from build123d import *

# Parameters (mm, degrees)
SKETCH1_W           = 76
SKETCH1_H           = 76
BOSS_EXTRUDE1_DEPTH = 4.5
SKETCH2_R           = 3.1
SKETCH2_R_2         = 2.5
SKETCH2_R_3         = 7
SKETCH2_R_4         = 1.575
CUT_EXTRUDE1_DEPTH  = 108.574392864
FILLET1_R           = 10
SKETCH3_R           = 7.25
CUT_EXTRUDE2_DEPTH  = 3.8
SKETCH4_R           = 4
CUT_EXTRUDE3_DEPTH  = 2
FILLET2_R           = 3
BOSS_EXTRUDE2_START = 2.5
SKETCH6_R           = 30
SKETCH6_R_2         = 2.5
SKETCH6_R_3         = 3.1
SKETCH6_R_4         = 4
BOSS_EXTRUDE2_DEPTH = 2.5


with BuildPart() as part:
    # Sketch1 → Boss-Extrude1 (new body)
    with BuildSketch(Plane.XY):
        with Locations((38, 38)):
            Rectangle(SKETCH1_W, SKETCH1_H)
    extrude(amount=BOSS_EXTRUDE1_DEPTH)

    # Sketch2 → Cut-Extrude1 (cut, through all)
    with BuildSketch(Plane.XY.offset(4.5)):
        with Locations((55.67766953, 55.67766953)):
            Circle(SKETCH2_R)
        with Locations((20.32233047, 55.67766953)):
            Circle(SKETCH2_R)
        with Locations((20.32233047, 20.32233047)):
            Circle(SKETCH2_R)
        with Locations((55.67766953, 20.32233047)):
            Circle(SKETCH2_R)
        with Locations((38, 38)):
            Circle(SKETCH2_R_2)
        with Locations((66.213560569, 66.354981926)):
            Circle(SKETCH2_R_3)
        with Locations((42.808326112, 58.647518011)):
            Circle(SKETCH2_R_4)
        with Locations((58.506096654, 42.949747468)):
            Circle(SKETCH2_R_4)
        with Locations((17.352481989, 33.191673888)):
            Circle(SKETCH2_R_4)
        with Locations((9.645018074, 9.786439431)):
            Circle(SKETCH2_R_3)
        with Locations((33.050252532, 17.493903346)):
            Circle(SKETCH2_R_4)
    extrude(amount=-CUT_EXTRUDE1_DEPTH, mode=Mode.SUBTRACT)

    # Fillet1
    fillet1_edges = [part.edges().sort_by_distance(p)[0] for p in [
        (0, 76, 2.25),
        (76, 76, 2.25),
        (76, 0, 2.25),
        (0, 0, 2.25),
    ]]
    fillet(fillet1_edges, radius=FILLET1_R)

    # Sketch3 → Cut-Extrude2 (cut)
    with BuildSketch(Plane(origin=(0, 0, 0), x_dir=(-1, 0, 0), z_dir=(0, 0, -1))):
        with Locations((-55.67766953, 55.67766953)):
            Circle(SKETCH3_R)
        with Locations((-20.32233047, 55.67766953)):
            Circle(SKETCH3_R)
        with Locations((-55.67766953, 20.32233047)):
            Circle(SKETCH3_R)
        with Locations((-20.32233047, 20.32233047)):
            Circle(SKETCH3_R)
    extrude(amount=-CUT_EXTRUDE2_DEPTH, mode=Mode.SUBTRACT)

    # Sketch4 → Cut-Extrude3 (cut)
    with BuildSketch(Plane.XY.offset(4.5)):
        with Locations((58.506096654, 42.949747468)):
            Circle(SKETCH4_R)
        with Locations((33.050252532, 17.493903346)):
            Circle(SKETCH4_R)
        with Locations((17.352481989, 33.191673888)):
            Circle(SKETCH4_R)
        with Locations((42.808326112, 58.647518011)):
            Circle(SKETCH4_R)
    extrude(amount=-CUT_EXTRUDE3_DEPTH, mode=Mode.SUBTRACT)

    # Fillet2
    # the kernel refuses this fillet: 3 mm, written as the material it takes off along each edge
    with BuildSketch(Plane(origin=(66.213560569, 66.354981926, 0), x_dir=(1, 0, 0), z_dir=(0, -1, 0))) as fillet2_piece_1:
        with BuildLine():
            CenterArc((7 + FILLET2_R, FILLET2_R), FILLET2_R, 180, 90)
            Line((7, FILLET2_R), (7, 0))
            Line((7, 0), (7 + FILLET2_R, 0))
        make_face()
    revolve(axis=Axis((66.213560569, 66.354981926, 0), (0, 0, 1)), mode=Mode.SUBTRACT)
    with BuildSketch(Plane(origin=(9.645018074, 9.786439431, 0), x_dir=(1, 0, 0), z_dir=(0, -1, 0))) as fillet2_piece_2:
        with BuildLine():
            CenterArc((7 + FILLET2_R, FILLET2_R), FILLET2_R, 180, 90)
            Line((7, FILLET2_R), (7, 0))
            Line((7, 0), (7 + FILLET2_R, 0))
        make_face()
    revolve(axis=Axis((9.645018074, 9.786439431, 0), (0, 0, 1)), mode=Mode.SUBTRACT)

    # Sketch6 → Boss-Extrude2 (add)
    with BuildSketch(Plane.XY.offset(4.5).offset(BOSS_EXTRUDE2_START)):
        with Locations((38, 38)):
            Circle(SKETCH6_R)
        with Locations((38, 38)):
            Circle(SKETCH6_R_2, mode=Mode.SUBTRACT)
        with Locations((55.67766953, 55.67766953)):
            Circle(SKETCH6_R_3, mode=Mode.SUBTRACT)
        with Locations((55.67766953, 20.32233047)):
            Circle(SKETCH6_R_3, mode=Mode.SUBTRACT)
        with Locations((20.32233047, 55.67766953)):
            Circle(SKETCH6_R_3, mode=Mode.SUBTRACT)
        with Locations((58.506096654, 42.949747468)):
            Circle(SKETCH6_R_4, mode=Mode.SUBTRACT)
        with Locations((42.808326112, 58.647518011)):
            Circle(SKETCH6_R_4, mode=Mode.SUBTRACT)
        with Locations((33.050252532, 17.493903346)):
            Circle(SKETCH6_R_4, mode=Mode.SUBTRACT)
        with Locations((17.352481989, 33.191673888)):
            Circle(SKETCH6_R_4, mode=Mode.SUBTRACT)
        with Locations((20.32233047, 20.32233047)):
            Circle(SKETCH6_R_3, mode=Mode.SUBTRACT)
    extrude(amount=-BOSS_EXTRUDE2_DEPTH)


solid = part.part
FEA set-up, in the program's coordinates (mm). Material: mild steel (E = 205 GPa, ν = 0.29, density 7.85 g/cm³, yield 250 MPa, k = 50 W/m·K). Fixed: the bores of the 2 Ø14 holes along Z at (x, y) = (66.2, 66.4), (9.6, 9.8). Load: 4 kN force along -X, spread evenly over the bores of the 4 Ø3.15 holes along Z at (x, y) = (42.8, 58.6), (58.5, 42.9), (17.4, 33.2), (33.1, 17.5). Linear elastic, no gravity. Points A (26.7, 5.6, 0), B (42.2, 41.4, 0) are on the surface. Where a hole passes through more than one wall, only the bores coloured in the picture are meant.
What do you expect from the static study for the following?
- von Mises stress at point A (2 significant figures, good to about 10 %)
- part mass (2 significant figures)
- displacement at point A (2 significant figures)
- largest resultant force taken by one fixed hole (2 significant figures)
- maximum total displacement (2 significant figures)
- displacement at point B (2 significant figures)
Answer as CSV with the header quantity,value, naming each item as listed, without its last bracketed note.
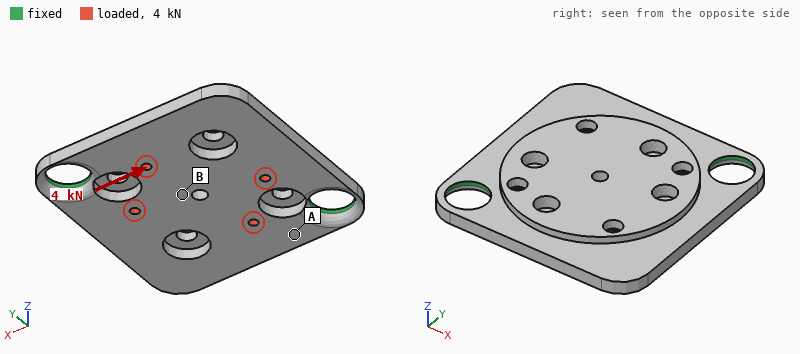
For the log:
quantity,value
von Mises stress at point A,19 MPa
part mass,210 g
displacement at point A,7.6 µm
largest resultant force taken by one fixed hole,2.0 kN
maximum total displacement,33 µm
displacement at point B,5.7 µm
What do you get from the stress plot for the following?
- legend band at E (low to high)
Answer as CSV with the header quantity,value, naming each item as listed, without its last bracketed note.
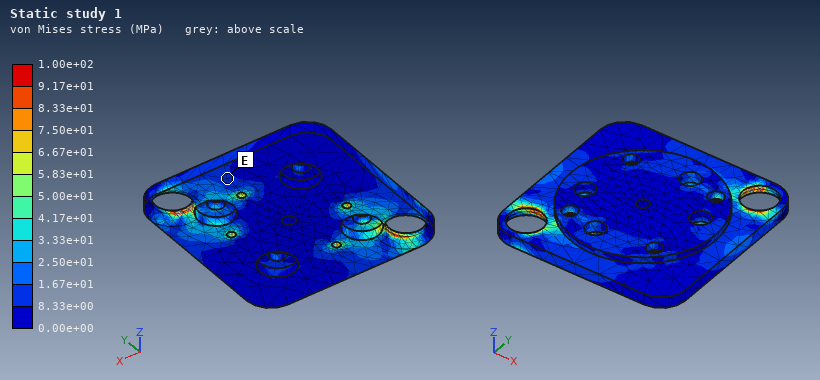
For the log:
quantity,value
legend band at E,8.33e+00 to 1.67e+01 MPa
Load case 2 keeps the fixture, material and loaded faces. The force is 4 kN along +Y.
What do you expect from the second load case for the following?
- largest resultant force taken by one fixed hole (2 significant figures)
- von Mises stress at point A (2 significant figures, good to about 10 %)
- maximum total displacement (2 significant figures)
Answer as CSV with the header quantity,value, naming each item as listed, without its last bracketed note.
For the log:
quantity,value
largest resultant force taken by one fixed hole,2.0 kN
von Mises stress at point A,19 MPa
maximum total displacement,33 µm
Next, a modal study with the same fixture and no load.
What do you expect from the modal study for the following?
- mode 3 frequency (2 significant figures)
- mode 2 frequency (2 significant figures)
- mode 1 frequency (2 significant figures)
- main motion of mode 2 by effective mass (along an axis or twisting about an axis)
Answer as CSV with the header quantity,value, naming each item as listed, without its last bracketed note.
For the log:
quantity,value
mode 3 frequency,6300 Hz
mode 2 frequency,2300 Hz
mode 1 frequency,1500 Hz
main motion of mode 2 by effective mass,along Z
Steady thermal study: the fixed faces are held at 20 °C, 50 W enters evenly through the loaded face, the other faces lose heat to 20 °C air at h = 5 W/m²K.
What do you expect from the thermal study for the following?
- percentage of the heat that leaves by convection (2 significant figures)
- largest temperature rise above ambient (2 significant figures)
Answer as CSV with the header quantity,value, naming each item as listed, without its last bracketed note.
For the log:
quantity,value
percentage of the heat that leaves by convection,7.3 %
largest temperature rise above ambient,86 K
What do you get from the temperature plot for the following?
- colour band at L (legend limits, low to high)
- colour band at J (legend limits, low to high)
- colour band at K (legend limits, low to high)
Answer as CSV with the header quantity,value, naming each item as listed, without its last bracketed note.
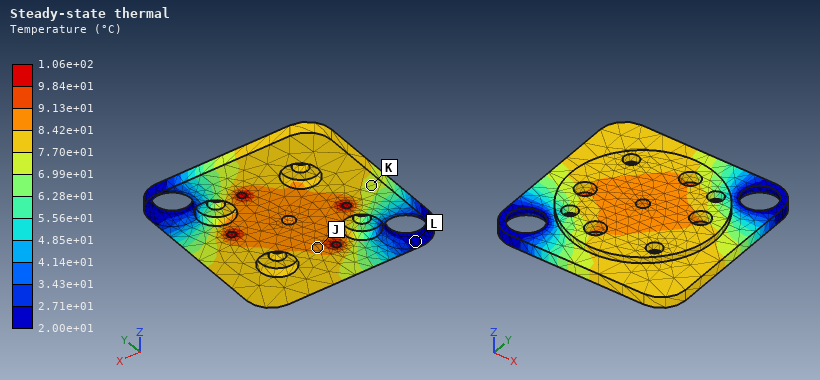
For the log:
quantity,value
colour band at L,2.00e+01 to 2.71e+01 °C
colour band at J,8.42e+01 to 9.13e+01 °C
colour band at K,6.99e+01 to 7.70e+01 °C
